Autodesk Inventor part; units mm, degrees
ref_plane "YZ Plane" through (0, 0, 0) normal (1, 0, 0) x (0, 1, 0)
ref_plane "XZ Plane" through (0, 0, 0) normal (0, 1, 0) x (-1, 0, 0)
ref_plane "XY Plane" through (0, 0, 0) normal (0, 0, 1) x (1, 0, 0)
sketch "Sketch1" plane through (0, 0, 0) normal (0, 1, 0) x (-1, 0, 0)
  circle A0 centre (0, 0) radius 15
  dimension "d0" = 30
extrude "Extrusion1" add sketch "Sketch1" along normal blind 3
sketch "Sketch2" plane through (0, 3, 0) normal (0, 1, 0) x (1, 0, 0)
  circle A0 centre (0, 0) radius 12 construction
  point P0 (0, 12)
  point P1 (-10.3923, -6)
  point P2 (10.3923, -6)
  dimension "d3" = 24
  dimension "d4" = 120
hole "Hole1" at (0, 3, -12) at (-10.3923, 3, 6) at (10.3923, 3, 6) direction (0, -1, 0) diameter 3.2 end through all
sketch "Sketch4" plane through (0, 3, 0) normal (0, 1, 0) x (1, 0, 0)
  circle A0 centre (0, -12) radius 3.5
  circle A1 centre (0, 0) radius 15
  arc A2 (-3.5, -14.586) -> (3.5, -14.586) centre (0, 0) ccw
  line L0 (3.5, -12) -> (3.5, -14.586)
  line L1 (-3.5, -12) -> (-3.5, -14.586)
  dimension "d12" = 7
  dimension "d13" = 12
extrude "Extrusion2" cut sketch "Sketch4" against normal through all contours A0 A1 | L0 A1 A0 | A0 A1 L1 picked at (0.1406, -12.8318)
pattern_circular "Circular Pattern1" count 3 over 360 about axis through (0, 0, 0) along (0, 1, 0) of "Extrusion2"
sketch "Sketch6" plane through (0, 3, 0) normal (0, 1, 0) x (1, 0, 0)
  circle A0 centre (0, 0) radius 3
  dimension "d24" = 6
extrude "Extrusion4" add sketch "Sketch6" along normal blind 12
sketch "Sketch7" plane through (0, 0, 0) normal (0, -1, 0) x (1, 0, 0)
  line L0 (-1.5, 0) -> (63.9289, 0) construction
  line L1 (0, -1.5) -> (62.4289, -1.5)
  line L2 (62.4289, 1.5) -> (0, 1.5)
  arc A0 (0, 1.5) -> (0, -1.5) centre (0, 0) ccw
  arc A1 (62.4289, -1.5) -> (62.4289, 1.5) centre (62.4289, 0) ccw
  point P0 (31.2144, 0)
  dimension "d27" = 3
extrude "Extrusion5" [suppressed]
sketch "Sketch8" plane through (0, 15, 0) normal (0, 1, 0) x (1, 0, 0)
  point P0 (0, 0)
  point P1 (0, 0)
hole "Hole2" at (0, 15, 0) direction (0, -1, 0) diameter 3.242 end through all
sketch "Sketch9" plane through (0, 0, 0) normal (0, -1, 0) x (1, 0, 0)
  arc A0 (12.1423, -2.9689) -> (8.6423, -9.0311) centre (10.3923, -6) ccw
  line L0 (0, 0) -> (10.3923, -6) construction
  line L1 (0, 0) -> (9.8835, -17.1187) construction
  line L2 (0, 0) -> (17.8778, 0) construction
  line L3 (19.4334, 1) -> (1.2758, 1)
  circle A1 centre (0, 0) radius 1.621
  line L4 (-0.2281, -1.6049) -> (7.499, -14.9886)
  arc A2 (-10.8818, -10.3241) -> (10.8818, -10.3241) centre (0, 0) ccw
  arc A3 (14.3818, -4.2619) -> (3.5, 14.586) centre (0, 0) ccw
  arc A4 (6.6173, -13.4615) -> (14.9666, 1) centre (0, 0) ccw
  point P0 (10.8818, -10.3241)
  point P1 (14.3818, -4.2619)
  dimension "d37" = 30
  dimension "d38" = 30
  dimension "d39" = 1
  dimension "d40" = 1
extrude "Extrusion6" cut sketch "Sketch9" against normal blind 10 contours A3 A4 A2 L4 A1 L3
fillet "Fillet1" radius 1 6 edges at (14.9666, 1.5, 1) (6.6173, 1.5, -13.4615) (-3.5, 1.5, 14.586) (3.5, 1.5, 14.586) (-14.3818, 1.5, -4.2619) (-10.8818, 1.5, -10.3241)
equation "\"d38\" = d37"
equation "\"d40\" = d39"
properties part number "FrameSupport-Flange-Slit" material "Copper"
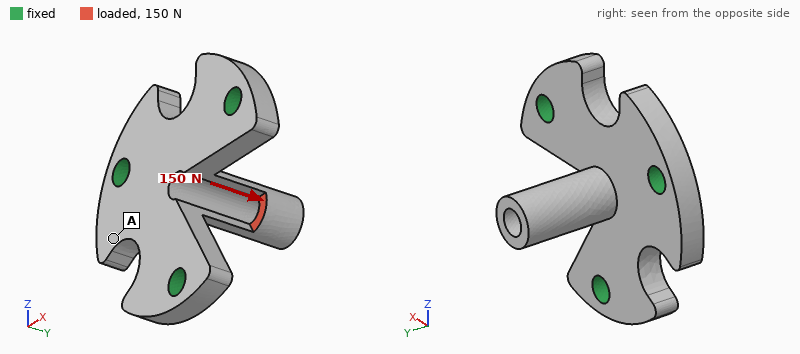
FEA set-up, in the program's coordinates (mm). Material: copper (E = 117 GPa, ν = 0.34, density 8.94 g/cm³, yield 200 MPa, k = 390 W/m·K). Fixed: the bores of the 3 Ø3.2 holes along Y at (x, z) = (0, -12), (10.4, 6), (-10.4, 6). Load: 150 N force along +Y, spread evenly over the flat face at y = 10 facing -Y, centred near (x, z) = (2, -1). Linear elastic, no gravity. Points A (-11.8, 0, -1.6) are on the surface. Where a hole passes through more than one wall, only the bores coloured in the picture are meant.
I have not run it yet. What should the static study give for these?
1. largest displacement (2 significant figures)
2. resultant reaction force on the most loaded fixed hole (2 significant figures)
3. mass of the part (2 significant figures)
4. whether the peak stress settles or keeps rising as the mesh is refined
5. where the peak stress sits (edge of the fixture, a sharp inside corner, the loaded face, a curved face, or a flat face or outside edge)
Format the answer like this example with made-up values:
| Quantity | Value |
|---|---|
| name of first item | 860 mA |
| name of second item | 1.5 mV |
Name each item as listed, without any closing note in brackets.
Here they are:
| Quantity | Value |
|---|---|
| largest displacement | 22 µm |
| resultant reaction force on the most loaded fixed hole | 61 N |
| mass of the part | 14 g |
| whether the peak stress settles or keeps rising as the mesh is refined | keeps rising |
| where the peak stress sits | a sharp inside corner |
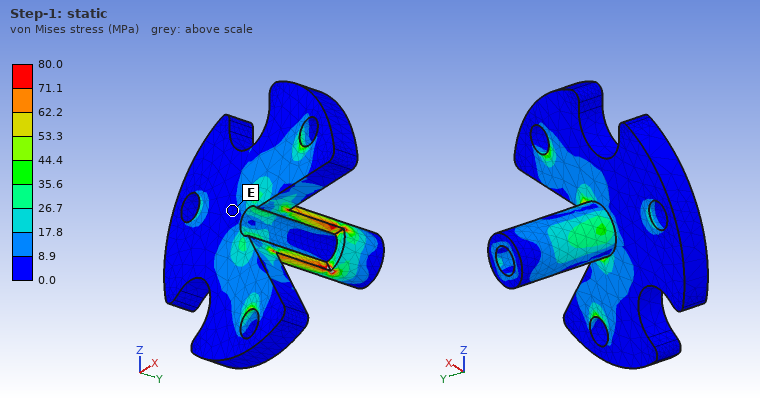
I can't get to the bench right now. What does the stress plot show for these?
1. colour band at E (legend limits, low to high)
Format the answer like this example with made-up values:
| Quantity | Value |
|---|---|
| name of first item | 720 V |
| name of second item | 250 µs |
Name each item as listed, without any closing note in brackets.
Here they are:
| Quantity | Value |
|---|---|
| colour band at E | 0.0 to 8.9 MPa |
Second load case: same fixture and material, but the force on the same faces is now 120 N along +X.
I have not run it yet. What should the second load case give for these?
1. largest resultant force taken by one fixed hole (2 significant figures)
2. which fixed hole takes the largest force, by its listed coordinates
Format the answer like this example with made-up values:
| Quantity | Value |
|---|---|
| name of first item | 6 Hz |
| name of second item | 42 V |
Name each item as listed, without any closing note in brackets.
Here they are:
| Quantity | Value |
|---|---|
| largest resultant force taken by one fixed hole | 84 N |
| which fixed hole takes the largest force, by its listed coordinates | (-10.4, 6) |
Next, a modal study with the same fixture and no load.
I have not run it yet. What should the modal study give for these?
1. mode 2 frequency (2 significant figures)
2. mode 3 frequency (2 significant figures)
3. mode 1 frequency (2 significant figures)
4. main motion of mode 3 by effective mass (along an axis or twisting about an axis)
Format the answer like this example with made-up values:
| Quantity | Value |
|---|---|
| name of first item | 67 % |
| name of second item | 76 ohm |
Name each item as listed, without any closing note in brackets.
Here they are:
| Quantity | Value |
|---|---|
| mode 2 frequency | 9900 Hz |
| mode 3 frequency | 20 kHz |
| mode 1 frequency | 9700 Hz |
| main motion of mode 3 by effective mass | along Y |
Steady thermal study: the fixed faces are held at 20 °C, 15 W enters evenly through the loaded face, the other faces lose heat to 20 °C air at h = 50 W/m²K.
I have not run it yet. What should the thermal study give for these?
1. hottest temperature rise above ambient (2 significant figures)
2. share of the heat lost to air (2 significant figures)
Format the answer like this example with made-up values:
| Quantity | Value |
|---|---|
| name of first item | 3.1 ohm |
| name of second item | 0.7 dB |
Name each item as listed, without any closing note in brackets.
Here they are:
| Quantity | Value |
|---|---|
| hottest temperature rise above ambient | 42 K |
| share of the heat lost to air | 3.1 % |
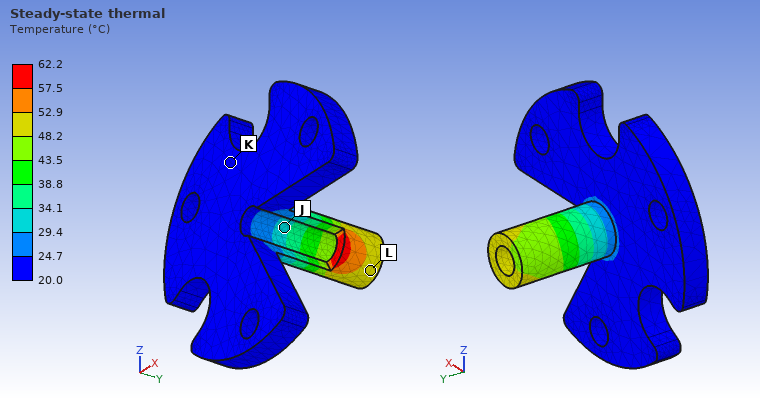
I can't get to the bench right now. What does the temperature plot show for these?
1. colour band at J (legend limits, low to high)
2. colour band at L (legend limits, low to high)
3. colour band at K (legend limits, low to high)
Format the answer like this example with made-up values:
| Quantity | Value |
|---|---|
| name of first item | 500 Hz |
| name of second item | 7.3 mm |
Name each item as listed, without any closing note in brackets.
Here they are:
| Quantity | Value |
|---|---|
| colour band at J | 29.4 to 34.1 °C |
| colour band at L | 48.2 to 52.9 °C |
| colour band at K | 20.0 to 24.7 °C |
